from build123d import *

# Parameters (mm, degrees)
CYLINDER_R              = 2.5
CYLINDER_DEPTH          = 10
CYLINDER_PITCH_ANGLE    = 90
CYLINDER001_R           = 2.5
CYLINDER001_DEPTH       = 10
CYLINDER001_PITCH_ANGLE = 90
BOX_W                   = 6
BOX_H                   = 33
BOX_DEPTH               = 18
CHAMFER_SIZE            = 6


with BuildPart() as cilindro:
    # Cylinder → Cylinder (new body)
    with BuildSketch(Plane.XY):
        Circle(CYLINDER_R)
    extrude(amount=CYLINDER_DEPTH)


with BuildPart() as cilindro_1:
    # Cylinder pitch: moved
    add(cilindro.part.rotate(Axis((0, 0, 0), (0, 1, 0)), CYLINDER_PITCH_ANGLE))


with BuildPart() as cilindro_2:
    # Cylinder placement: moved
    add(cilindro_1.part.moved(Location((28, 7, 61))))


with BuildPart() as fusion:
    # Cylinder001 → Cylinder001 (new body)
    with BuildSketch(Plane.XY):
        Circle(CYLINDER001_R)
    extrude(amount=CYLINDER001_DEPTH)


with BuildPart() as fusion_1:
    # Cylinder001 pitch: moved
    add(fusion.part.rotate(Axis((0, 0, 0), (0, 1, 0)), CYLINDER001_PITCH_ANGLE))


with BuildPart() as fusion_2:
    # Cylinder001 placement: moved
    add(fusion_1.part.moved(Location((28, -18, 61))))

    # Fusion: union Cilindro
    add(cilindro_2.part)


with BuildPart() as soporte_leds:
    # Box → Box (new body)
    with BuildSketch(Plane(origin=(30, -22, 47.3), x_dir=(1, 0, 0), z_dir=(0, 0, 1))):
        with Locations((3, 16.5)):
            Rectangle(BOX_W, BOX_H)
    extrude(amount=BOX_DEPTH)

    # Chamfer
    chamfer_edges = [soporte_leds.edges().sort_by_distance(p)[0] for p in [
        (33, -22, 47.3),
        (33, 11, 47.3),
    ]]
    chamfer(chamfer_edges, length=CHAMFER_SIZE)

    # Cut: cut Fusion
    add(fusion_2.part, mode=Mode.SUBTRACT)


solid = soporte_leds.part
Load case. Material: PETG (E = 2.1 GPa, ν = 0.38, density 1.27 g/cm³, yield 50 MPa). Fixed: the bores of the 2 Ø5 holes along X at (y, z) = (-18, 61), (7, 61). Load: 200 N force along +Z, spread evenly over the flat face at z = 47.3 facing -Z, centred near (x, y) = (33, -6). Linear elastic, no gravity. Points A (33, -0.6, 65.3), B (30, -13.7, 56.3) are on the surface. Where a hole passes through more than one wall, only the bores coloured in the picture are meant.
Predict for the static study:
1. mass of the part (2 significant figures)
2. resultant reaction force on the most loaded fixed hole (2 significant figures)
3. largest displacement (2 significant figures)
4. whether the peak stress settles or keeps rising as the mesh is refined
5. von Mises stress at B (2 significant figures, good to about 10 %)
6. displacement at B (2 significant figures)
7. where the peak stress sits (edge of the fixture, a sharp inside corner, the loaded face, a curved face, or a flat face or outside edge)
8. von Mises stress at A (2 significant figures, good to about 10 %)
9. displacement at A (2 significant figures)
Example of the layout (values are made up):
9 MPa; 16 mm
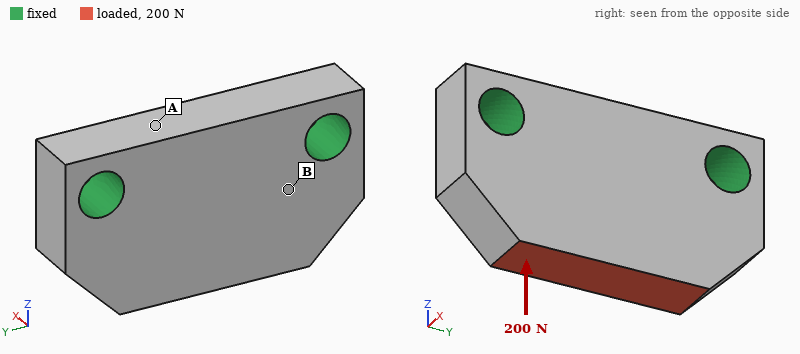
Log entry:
4.0 g; 110 N; 16 µm; keeps rising; 2.1 MPa; 5.8 µm; edge of the fixture; 0.80 MPa; 8.0 µm
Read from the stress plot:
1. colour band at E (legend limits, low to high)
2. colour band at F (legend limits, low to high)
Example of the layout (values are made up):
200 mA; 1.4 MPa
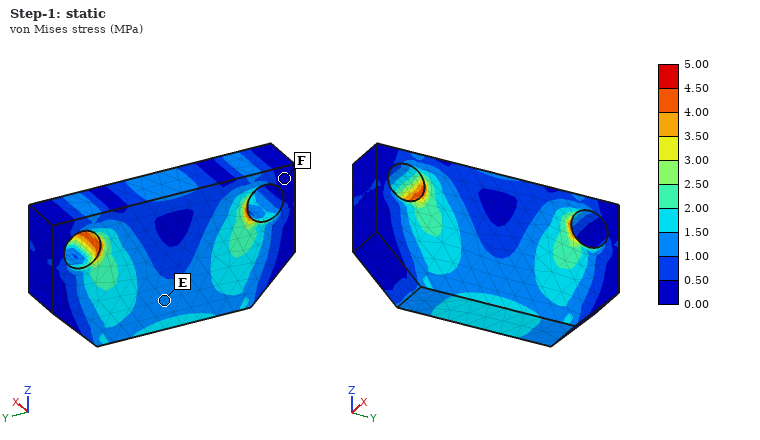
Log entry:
1.00 to 1.50 MPa; 0.00 to 0.50 MPa
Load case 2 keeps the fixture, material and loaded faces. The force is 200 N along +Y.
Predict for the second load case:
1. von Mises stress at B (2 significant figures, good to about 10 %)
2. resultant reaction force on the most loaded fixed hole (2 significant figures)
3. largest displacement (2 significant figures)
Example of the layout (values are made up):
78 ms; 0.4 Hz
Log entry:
2.3 MPa; 140 N; 25 µm
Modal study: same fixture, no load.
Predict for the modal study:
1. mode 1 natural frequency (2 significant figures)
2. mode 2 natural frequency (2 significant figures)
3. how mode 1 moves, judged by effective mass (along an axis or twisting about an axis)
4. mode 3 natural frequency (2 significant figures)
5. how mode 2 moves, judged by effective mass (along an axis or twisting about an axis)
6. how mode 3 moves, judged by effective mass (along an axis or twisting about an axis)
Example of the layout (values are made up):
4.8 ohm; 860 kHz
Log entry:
5700 Hz; 11 kHz; along X; 12 kHz; twisting about Z; along X
